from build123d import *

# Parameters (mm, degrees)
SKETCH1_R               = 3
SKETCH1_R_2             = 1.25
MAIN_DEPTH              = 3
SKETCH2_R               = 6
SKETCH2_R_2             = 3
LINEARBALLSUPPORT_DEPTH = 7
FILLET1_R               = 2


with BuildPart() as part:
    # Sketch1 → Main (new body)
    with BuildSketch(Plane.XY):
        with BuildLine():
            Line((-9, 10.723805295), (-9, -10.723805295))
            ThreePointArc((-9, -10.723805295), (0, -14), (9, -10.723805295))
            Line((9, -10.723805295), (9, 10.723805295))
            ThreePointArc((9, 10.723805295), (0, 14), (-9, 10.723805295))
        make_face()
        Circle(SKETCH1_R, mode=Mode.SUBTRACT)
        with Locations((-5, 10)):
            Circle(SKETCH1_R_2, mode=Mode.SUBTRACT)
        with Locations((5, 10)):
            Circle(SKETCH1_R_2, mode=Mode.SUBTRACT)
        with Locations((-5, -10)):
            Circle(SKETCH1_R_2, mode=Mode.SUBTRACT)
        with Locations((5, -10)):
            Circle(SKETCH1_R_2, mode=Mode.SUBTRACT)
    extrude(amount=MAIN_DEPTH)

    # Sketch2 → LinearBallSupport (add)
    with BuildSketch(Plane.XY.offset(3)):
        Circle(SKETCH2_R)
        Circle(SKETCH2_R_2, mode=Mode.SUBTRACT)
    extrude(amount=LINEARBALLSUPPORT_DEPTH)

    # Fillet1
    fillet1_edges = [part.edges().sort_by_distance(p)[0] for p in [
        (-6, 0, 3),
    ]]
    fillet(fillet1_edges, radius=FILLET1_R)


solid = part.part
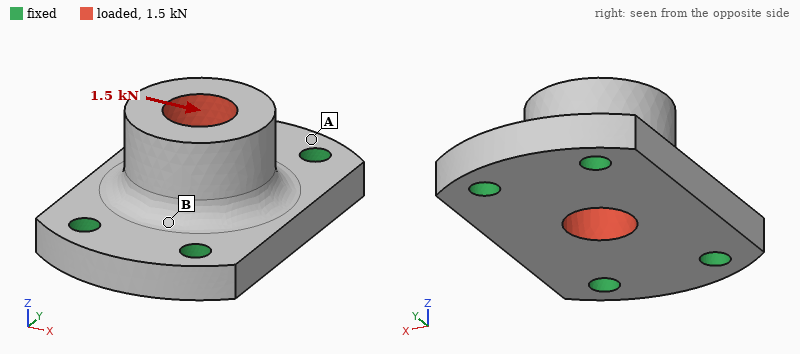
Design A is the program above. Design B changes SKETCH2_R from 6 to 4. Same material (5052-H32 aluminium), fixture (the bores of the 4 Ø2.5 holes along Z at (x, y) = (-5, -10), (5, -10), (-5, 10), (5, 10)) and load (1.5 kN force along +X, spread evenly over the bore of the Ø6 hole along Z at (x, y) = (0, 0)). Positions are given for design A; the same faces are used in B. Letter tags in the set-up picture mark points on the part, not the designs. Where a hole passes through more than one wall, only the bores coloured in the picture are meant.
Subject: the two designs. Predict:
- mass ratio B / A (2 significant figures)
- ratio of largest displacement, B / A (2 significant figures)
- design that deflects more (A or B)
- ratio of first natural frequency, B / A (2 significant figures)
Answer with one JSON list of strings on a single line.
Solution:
["0.76", "2.2", "B", "1.2"]
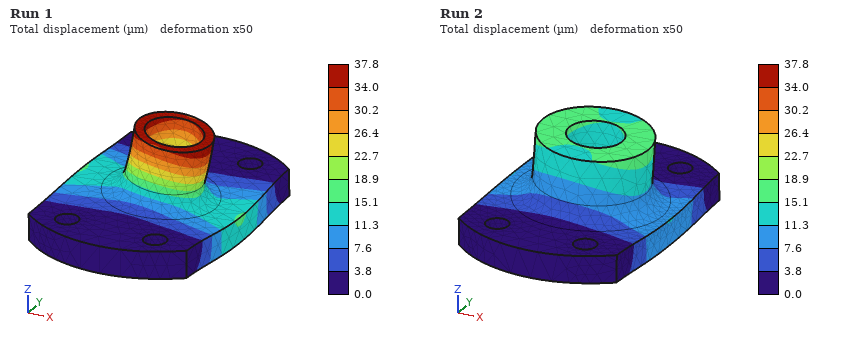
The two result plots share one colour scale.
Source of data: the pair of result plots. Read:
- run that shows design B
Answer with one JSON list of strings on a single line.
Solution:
["Run 1"]
